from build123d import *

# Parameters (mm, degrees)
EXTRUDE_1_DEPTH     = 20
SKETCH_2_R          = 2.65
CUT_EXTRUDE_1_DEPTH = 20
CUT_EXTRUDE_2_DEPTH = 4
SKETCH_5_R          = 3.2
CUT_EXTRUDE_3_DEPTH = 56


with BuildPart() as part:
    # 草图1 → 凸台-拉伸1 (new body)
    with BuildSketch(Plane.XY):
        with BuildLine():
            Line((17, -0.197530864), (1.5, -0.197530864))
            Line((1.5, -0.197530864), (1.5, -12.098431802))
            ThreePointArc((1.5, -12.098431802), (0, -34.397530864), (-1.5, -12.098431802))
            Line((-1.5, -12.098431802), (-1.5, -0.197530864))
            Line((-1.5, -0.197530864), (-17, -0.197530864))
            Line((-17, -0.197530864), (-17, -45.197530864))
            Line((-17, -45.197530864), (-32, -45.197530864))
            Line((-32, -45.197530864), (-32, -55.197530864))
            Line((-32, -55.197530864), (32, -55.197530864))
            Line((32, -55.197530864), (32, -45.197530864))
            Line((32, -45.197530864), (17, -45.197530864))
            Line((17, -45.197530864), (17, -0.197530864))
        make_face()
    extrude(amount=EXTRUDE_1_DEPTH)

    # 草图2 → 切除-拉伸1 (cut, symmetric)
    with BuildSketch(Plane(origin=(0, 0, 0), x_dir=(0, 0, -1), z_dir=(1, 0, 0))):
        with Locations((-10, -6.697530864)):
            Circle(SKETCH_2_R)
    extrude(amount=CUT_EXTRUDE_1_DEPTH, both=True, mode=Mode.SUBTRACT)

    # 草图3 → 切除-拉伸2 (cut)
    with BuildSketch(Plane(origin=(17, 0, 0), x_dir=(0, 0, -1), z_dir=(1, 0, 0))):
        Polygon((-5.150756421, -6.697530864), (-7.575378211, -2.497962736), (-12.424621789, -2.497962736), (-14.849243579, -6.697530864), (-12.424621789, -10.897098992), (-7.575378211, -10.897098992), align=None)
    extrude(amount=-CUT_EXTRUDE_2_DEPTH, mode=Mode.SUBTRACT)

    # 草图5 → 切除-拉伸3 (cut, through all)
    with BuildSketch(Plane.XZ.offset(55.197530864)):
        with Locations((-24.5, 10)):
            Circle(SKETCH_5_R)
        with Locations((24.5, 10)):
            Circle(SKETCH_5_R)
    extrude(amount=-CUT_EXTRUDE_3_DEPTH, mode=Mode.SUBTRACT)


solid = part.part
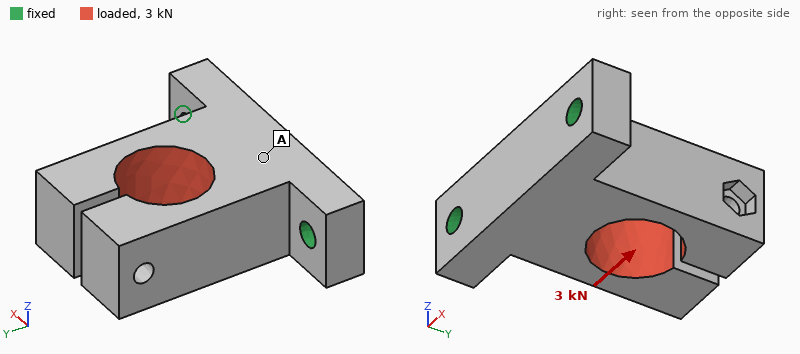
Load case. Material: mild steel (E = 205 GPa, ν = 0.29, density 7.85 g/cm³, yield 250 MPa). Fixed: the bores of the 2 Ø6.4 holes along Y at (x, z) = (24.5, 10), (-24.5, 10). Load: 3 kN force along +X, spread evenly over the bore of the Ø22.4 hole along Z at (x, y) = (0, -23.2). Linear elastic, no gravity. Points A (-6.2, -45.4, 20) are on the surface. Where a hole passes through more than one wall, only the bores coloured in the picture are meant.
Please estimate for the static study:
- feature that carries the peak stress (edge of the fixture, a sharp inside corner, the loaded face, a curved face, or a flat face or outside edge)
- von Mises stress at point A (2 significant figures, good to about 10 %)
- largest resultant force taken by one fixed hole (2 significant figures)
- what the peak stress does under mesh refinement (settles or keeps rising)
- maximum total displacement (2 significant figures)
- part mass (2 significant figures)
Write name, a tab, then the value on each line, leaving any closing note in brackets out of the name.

feature that carries the peak stress	edge of the fixture
von Mises stress at point A	11 MPa
largest resultant force taken by one fixed hole	2.5 kN
what the peak stress does under mesh refinement	keeps rising
maximum total displacement	45 µm
part mass	260 g
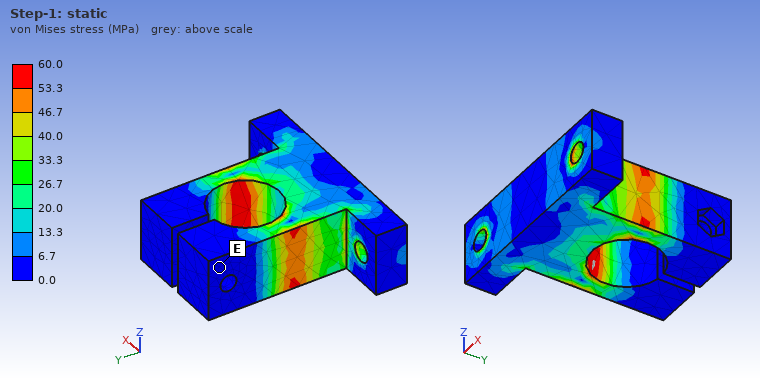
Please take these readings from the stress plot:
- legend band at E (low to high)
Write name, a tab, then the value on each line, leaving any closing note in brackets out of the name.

legend band at E	0.0 to 6.7 MPa
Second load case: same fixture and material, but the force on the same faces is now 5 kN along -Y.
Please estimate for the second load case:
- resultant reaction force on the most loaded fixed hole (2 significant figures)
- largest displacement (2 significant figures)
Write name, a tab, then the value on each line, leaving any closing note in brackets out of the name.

resultant reaction force on the most loaded fixed hole	2.7 kN
largest displacement	43 µm
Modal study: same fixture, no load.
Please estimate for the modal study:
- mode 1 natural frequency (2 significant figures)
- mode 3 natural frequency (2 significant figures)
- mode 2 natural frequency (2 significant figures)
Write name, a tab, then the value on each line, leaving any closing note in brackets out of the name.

mode 1 natural frequency	3100 Hz
mode 3 natural frequency	3200 Hz
mode 2 natural frequency	3100 Hz
